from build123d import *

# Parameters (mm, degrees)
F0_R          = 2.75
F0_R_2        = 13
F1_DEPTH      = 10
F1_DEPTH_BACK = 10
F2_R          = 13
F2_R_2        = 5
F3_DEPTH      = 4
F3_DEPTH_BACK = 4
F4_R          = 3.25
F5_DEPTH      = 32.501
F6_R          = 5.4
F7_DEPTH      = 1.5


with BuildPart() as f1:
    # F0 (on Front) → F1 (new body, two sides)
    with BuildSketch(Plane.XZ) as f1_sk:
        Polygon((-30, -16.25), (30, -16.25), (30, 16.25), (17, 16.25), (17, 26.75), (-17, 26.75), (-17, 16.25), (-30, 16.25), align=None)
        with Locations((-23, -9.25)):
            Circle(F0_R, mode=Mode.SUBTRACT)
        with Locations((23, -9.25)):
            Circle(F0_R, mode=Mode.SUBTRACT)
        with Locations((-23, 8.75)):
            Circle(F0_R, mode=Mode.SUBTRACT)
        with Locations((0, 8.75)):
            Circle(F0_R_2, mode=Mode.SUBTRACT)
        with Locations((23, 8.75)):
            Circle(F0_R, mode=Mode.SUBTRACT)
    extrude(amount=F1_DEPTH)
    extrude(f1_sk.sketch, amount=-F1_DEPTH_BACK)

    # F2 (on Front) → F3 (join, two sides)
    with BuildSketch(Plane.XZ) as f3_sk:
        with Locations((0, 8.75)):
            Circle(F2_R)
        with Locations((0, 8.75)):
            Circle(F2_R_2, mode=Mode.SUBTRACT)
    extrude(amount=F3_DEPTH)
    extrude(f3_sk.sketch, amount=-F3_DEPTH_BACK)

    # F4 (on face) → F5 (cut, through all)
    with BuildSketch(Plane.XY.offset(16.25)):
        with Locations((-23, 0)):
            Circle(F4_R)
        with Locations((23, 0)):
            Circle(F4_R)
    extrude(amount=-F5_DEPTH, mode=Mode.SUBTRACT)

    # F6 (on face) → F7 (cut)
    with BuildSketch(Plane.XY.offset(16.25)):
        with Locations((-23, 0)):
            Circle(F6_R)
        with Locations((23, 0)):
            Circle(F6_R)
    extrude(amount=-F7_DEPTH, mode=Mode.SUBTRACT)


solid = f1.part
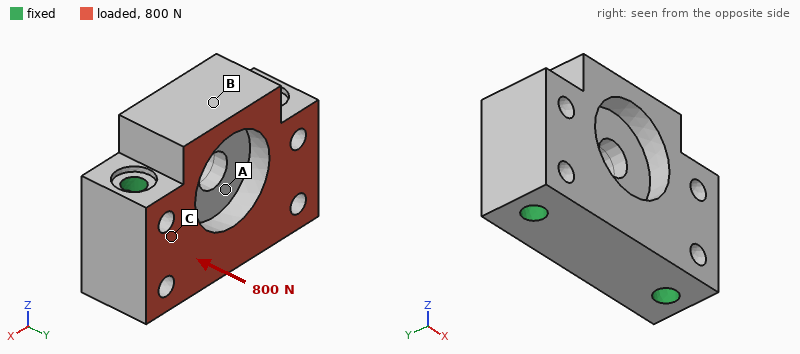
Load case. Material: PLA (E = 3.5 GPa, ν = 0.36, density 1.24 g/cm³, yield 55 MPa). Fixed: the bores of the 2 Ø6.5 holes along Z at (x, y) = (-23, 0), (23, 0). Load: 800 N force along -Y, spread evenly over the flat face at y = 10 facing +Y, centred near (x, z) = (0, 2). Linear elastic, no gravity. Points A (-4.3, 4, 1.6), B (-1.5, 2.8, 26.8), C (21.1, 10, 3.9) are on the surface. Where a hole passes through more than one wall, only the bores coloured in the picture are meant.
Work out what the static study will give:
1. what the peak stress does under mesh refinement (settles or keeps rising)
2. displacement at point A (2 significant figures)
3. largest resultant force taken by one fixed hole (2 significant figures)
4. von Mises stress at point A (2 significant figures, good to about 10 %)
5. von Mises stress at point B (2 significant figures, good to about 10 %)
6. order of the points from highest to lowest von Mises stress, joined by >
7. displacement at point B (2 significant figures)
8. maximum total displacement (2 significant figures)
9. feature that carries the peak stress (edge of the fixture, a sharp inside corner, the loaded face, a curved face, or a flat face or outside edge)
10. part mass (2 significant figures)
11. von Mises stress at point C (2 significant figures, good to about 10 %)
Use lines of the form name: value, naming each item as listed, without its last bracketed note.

what the peak stress does under mesh refinement: keeps rising
displacement at point A: 7.4 µm
largest resultant force taken by one fixed hole: 400 N
von Mises stress at point A: 0.67 MPa
von Mises stress at point B: 0.39 MPa
order of the points from highest to lowest von Mises stress, joined by >: C > A > B
displacement at point B: 24 µm
maximum total displacement: 26 µm
feature that carries the peak stress: edge of the fixture
part mass: 44 g
von Mises stress at point C: 1.3 MPa
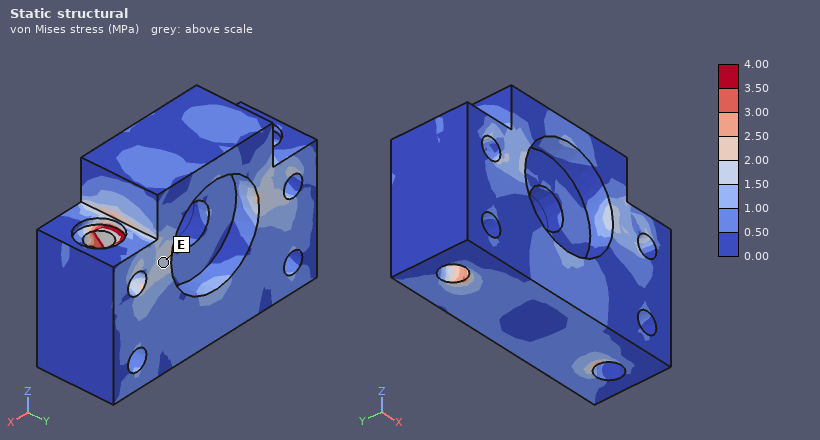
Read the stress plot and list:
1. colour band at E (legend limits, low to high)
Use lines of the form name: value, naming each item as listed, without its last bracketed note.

colour band at E: 1.50 to 2.00 MPa
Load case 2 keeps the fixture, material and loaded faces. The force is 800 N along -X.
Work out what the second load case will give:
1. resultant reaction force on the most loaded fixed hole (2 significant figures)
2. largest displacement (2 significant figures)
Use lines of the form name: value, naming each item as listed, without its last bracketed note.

resultant reaction force on the most loaded fixed hole: 420 N
largest displacement: 15 µm
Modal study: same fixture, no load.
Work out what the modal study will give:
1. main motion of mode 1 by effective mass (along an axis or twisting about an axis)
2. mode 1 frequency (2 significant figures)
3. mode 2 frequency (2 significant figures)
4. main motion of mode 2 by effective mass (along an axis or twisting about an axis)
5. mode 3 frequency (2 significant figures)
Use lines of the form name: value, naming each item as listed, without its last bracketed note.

main motion of mode 1 by effective mass: along Y
mode 1 frequency: 5000 Hz
mode 2 frequency: 8100 Hz
main motion of mode 2 by effective mass: along Y
mode 3 frequency: 8800 Hz
